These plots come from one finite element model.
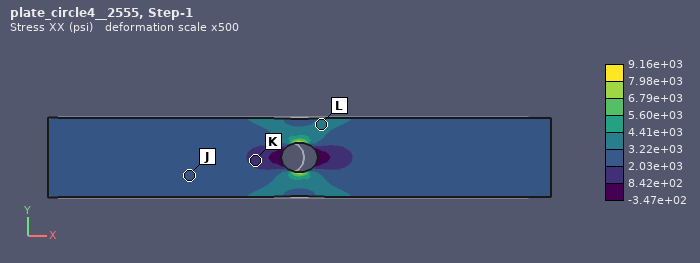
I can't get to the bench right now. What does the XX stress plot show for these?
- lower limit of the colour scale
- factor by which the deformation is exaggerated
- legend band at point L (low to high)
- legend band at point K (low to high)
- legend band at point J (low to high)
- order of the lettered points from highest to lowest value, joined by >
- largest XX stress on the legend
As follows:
-3.47e+02 psi
500
3.22e+03 to 4.41e+03 psi
8.42e+02 to 2.03e+03 psi
2.03e+03 to 3.22e+03 psi
L > J > K
9.16e+03 psi
